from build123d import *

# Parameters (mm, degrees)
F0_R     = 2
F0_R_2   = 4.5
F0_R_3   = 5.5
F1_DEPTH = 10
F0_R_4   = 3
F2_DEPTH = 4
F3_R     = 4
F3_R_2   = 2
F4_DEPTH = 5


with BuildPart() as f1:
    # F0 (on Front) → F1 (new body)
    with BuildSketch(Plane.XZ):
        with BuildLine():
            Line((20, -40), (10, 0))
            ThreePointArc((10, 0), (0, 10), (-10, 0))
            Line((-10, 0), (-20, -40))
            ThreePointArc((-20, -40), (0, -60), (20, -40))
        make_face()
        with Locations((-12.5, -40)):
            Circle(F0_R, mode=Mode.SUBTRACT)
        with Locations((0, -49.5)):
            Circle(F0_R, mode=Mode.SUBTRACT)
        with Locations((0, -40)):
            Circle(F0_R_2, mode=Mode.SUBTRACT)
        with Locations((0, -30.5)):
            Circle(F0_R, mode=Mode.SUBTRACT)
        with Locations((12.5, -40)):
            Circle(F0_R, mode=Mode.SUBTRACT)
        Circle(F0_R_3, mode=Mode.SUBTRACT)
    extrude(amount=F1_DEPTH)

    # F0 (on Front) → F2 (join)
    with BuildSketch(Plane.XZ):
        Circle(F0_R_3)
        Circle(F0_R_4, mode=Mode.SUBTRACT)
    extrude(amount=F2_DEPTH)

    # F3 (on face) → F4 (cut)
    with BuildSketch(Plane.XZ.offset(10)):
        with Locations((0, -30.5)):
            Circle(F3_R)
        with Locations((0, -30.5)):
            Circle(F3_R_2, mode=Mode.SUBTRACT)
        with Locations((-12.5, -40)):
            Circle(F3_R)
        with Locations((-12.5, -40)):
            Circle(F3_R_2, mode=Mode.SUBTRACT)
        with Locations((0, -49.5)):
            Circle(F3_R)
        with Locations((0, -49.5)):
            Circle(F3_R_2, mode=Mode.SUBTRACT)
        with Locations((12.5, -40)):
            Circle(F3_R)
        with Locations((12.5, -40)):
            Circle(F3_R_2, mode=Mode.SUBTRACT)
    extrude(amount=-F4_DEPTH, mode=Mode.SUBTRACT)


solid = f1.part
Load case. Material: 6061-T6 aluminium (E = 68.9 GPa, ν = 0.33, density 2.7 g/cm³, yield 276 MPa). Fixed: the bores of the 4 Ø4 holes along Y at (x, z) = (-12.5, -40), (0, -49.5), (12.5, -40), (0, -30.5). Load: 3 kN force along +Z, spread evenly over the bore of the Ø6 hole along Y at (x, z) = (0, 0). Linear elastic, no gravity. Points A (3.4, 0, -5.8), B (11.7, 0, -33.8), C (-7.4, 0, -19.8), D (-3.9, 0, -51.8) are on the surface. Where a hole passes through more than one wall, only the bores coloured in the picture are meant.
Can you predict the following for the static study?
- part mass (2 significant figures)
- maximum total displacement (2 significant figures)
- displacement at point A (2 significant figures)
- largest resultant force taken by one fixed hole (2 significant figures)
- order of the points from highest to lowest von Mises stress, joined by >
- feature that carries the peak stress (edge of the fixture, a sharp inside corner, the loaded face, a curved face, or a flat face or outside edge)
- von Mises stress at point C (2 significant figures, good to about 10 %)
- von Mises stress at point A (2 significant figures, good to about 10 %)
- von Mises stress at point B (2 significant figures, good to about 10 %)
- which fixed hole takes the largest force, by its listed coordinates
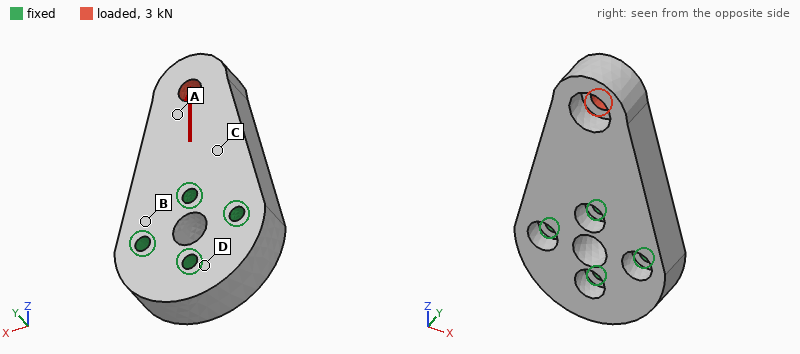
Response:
47 g
50 µm
22 µm
1.6 kN
A > C > B > D
the loaded face
28 MPa
45 MPa
18 MPa
(0, -30.5)
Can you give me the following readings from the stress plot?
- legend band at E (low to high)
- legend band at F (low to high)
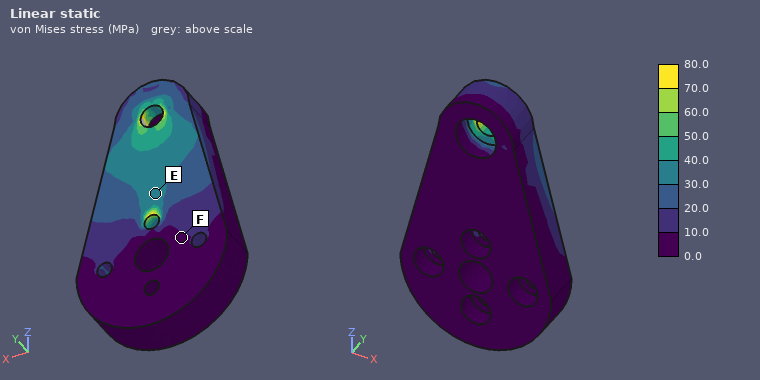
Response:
30.0 to 40.0 MPa
0.0 to 10.0 MPa
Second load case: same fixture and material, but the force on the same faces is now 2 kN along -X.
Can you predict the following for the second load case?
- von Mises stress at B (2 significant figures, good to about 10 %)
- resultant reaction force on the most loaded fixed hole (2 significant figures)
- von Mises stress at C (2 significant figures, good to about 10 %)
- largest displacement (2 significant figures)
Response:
32 MPa
2.0 kN
26 MPa
52 µm
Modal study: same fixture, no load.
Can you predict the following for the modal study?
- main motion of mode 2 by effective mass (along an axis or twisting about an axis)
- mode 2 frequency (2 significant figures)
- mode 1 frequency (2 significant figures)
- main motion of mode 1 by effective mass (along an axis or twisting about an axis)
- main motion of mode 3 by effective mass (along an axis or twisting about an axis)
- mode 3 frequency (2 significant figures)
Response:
along X
12 kHz
5100 Hz
along Y
twisting about Z
14 kHz
